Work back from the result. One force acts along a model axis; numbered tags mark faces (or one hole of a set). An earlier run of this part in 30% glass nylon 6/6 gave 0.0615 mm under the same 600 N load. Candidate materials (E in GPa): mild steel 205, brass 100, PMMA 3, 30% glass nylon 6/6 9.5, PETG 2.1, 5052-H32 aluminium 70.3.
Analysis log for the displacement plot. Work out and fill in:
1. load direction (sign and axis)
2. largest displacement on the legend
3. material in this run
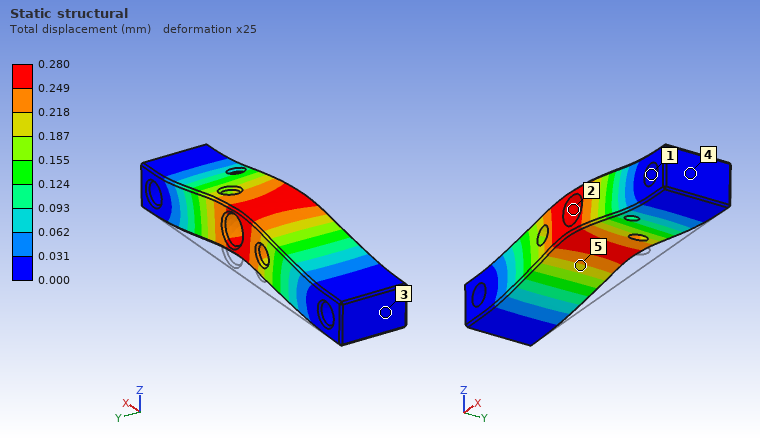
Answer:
+Z
0.280 mm
PETG
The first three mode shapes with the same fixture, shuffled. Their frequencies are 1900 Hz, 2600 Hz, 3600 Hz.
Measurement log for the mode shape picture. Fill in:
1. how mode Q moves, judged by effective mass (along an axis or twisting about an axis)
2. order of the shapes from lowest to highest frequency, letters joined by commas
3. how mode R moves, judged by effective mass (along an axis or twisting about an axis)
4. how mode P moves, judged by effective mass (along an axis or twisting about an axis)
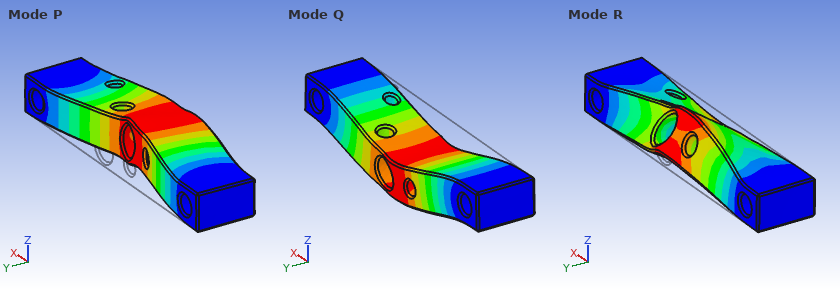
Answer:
along Z
Q, P, R
twisting about X
along Y
